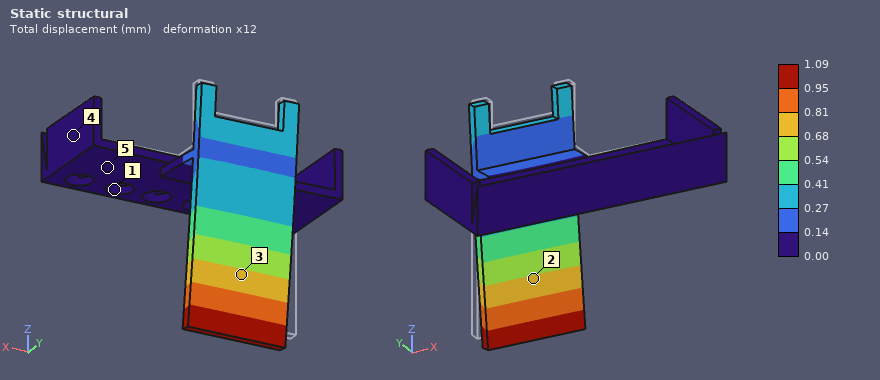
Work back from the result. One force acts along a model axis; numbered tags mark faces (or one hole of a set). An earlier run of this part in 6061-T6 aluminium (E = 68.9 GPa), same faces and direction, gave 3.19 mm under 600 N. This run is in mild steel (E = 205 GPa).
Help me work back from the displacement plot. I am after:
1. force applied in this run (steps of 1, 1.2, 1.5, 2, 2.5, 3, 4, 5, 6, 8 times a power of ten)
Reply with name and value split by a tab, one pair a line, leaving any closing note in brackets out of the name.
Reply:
force applied in this run	600 N
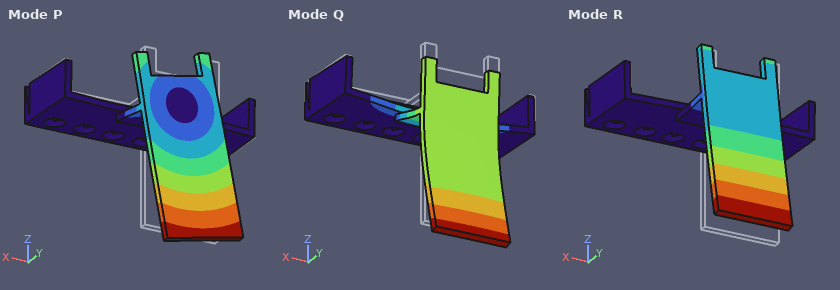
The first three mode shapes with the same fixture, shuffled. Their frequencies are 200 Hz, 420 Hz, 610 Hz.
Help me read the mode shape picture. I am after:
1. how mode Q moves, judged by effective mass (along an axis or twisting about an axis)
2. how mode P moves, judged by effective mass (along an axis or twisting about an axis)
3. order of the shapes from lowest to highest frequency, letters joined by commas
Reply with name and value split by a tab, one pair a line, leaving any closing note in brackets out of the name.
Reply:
how mode Q moves, judged by effective mass	along Z
how mode P moves, judged by effective mass	along X
order of the shapes from lowest to highest frequency, letters joined by commas	R, P, Q
